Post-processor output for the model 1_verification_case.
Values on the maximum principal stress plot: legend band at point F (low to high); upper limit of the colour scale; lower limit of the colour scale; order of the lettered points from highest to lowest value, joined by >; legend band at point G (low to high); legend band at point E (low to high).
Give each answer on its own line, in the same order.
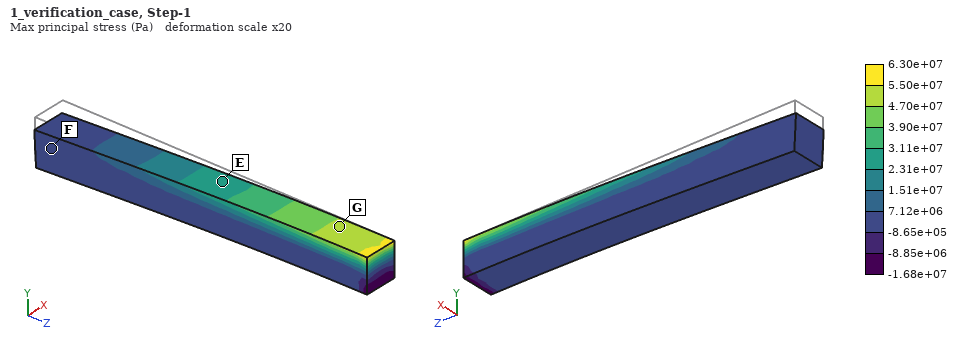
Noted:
-8.65e+05 to 7.12e+06 Pa
6.30e+07 Pa
-1.68e+07 Pa
G > E > F
4.70e+07 to 5.50e+07 Pa
2.31e+07 to 3.11e+07 Pa
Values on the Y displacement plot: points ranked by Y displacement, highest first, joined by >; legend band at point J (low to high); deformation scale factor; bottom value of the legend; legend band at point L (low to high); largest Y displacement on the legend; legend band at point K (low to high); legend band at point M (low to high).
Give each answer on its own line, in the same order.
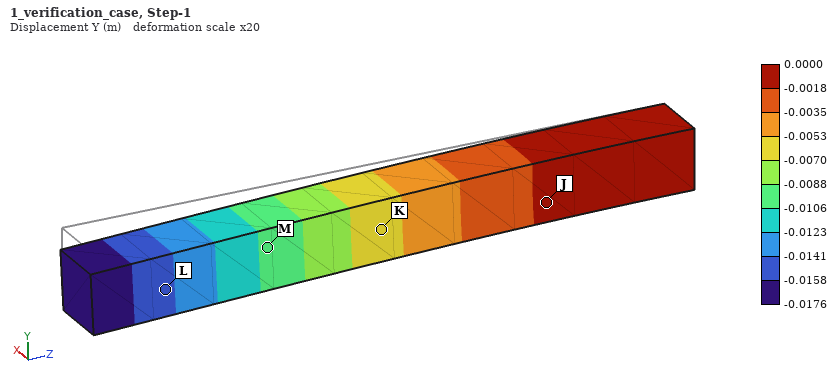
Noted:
J > K > M > L
-0.0018 to 0.0000 m
20
-0.0176 m
-0.0158 to -0.0141 m
0.0000 m
-0.0070 to -0.0053 m
-0.0106 to -0.0088 m
